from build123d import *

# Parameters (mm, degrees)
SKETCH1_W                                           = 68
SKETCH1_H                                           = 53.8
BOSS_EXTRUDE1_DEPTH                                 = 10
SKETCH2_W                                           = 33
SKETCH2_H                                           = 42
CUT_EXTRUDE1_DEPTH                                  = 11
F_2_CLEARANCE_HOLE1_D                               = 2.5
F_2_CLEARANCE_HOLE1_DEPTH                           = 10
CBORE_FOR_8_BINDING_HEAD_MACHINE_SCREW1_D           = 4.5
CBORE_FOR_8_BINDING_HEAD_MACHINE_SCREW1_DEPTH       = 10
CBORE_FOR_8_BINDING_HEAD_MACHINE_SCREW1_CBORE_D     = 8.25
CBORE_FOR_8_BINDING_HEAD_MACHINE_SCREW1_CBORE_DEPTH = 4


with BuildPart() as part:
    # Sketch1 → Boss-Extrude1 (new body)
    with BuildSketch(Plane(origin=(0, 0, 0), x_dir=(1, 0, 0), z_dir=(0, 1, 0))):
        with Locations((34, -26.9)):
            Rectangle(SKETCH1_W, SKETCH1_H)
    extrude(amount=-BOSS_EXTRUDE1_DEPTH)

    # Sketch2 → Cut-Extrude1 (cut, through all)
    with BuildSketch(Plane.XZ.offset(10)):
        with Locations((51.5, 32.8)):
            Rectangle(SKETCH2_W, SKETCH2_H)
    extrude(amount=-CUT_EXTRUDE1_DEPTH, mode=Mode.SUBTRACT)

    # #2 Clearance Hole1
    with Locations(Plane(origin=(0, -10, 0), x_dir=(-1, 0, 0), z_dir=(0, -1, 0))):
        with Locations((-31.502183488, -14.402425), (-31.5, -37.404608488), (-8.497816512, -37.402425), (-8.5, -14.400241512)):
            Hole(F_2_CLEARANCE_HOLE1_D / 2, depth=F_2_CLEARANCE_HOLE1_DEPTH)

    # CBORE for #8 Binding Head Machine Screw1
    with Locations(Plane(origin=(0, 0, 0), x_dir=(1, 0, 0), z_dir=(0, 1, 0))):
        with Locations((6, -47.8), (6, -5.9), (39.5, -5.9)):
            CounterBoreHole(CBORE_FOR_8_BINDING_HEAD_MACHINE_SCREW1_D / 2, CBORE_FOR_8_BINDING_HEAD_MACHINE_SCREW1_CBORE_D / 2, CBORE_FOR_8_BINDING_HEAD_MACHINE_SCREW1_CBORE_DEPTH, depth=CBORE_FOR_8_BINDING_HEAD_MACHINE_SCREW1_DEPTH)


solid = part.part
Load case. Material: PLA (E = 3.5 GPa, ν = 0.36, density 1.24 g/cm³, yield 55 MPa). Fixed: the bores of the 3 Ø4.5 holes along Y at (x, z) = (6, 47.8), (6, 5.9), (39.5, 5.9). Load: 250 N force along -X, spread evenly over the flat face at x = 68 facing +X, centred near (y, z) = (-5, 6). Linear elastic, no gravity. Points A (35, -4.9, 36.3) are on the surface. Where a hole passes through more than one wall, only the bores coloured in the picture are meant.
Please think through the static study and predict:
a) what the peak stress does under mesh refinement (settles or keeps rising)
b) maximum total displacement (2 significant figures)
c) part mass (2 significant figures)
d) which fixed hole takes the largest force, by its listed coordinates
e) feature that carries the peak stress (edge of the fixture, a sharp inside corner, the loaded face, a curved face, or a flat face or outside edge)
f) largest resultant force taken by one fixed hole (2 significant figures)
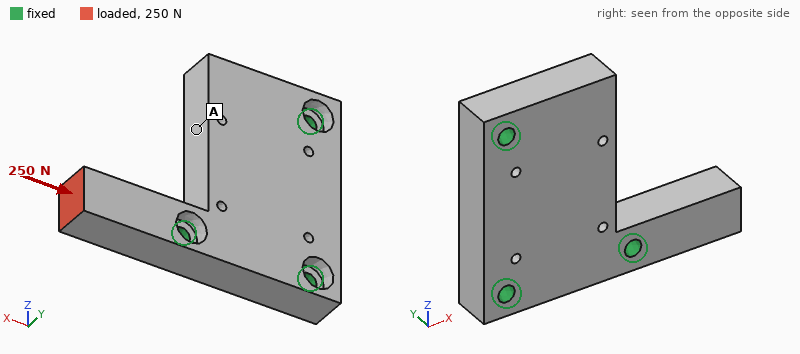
keeps rising
45 µm
27 g
(39.5, 5.9)
edge of the fixture
220 N
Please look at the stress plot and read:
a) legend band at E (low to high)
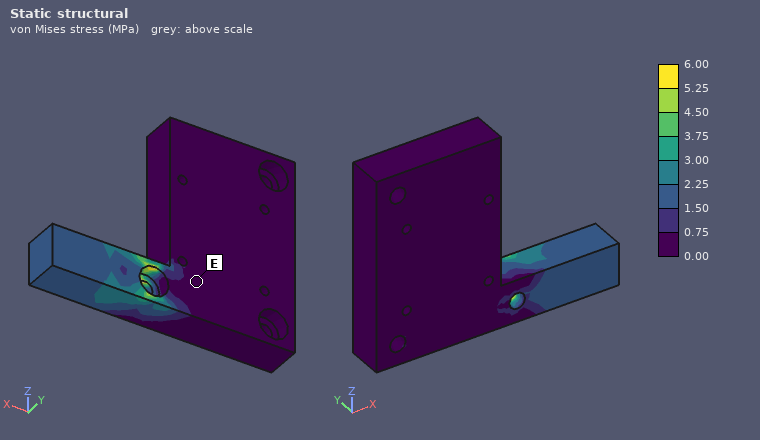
0.00 to 0.75 MPa
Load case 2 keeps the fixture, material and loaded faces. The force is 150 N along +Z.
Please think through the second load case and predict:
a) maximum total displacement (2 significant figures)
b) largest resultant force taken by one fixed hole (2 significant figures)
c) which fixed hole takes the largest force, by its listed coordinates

0.40 mm
240 N
(39.5, 5.9)
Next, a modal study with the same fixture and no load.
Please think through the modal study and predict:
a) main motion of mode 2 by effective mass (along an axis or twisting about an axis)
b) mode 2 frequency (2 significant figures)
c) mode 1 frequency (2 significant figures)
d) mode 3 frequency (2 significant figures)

along Y
2700 Hz
2400 Hz
2900 Hz
